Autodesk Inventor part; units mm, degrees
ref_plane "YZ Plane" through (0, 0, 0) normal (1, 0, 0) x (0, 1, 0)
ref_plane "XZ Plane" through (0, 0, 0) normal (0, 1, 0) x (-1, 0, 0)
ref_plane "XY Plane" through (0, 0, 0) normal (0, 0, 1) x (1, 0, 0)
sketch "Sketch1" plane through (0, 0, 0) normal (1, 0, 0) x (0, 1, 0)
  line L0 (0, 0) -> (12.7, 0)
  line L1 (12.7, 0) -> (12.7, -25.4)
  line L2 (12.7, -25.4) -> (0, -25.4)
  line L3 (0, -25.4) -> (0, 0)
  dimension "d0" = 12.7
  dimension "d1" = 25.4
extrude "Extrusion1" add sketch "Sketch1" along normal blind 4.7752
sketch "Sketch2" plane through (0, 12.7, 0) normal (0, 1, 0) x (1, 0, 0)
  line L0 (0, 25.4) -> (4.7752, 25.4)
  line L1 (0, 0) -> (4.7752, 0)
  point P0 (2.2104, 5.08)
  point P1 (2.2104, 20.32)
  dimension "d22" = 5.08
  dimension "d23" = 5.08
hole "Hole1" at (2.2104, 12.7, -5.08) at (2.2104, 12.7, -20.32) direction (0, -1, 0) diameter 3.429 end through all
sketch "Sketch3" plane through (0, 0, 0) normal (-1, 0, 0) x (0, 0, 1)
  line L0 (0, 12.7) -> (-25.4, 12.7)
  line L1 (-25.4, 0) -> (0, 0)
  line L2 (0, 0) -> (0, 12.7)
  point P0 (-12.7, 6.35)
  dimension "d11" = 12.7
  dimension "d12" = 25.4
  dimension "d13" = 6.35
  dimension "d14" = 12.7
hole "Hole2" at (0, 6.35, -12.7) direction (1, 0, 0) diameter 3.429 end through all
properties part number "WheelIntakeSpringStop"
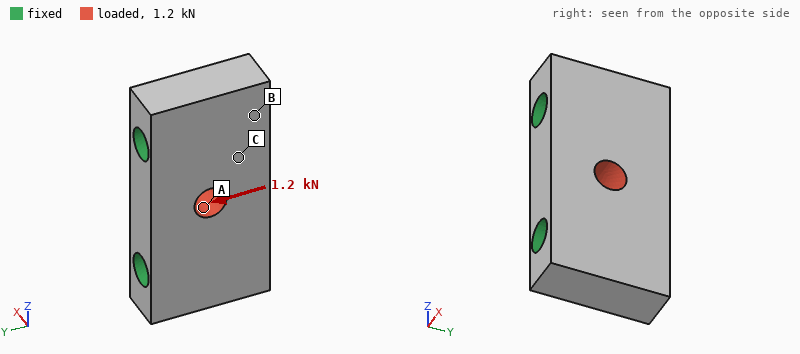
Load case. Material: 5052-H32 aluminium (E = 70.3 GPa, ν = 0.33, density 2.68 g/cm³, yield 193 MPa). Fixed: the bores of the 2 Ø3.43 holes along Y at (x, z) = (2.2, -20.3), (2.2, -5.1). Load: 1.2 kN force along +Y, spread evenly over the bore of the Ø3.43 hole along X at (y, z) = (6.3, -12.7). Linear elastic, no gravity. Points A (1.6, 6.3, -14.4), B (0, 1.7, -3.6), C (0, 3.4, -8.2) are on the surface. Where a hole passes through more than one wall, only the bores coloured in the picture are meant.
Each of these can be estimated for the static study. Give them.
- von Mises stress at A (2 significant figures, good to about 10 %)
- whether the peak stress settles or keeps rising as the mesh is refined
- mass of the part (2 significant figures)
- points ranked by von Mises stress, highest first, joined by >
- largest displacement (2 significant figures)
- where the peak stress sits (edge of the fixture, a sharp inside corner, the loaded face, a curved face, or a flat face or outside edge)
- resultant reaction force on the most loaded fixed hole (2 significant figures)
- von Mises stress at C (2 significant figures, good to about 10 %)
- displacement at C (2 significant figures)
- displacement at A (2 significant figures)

41 MPa
keeps rising
3.4 g
A > C > B
2.8 µm
edge of the fixture
600 N
19 MPa
0.74 µm
2.4 µm
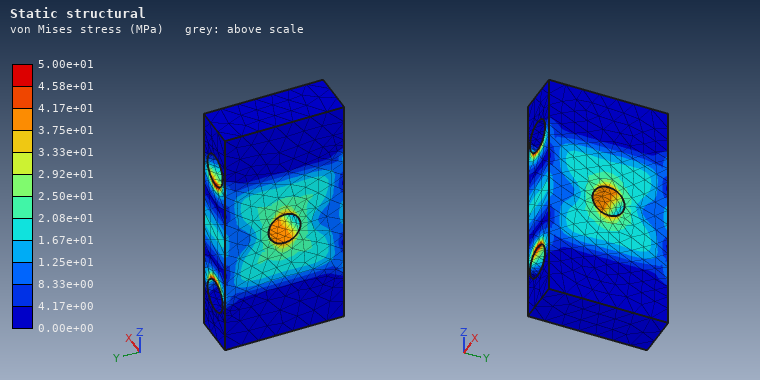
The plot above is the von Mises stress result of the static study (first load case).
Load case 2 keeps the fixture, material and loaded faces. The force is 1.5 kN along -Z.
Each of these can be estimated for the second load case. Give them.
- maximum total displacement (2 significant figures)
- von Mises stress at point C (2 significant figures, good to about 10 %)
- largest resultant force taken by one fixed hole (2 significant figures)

1.7 µm
13 MPa
750 N
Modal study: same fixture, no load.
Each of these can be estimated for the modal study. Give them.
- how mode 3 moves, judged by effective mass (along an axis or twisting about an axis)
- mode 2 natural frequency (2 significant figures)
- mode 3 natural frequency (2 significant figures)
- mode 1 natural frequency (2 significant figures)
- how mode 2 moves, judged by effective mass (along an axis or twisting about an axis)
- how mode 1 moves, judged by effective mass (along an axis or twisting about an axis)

along Y
99 kHz
120 kHz
90 kHz
twisting about Z
along X
